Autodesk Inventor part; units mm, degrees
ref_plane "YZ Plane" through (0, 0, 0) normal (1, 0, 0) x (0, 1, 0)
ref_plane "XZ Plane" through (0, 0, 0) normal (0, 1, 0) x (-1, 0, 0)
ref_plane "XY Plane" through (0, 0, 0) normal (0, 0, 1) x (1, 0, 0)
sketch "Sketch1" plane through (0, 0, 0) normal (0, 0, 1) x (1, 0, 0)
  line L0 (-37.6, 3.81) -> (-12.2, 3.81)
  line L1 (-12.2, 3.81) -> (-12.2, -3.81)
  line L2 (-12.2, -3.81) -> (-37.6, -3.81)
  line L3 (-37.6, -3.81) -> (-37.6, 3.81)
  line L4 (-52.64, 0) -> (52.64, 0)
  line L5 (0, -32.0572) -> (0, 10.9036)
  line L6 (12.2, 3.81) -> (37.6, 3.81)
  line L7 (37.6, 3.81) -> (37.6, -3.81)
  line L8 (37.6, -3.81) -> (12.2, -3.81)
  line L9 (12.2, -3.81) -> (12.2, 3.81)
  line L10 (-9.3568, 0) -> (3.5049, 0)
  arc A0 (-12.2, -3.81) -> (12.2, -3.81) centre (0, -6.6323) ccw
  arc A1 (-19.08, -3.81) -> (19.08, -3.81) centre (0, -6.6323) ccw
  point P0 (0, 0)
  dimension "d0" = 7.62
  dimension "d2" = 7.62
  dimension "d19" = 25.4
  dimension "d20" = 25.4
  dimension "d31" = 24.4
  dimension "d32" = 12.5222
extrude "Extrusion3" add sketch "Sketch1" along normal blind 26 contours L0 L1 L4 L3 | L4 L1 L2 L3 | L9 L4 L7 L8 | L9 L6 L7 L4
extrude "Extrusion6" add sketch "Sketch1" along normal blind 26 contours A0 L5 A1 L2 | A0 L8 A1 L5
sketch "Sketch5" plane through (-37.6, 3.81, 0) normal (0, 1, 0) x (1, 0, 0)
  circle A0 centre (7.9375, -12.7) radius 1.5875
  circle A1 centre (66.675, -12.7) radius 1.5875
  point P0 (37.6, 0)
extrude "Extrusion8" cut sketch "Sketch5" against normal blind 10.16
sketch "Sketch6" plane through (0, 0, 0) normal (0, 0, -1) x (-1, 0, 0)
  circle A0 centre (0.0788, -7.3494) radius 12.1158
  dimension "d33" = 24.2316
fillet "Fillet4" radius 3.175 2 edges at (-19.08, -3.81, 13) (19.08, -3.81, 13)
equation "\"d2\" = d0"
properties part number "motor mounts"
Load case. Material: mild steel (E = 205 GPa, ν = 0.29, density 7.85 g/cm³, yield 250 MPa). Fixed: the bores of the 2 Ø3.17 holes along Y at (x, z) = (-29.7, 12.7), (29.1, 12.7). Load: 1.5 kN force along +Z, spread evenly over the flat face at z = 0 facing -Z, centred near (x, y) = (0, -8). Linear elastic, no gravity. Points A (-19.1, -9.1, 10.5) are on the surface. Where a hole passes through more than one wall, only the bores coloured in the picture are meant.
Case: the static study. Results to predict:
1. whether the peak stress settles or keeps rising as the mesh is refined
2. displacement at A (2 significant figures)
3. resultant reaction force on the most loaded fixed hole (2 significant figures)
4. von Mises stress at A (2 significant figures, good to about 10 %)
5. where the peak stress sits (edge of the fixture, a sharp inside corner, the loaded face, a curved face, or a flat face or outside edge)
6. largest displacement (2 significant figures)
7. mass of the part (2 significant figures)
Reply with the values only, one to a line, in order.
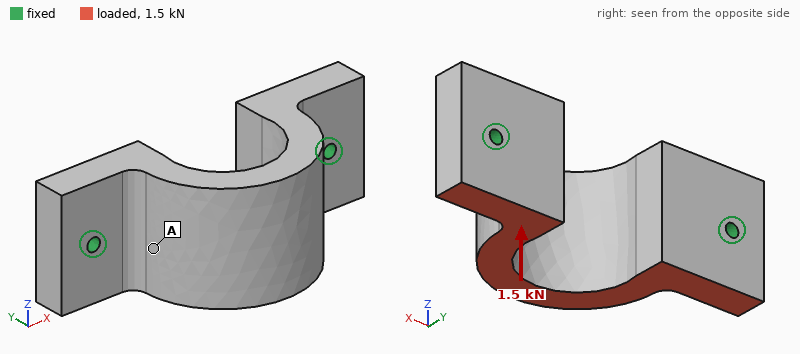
keeps rising
6.6 µm
760 N
15 MPa
edge of the fixture
16 µm
160 g
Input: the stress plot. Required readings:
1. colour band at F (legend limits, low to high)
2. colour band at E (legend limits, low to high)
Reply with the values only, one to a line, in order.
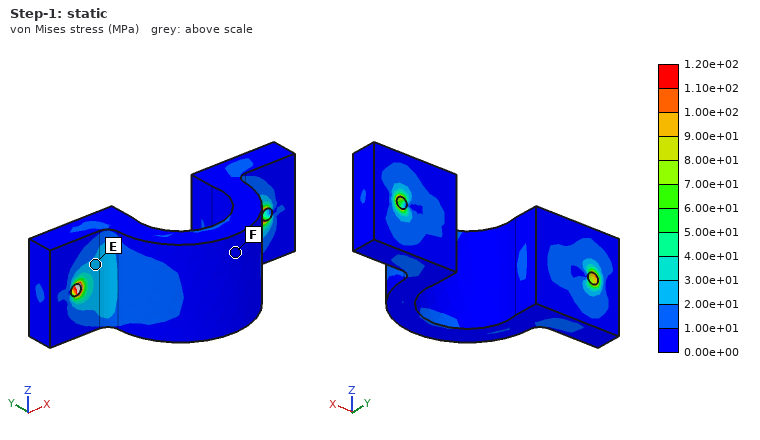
0.00e+00 to 1.00e+01 MPa
2.00e+01 to 3.00e+01 MPa
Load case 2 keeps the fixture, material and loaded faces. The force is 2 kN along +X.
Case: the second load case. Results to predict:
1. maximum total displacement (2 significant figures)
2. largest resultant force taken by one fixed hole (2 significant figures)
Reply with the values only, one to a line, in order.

6.7 µm
1.1 kN
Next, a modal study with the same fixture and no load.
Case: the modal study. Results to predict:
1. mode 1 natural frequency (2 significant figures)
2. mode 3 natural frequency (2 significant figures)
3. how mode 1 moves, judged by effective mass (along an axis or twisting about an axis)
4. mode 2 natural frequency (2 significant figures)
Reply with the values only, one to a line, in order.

4500 Hz
11 kHz
along Z
11 kHz
